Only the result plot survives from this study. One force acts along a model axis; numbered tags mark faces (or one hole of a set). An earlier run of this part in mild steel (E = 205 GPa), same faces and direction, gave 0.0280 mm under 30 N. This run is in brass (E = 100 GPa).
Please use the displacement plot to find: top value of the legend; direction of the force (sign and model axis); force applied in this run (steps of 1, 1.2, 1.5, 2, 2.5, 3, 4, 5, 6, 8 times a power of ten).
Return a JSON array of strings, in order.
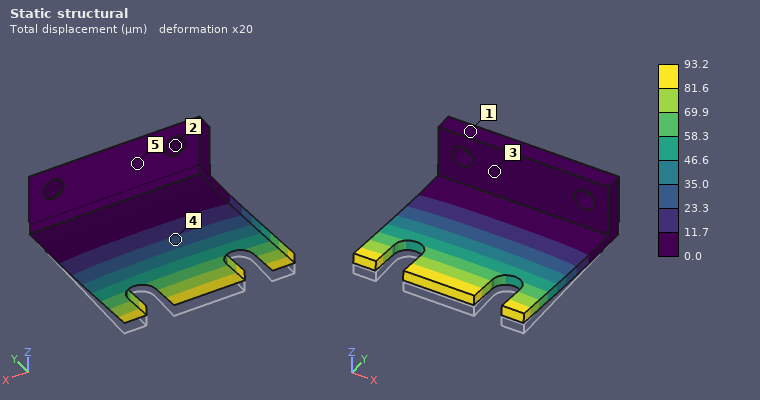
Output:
["93.2 µm", "+Z", "50 N"]
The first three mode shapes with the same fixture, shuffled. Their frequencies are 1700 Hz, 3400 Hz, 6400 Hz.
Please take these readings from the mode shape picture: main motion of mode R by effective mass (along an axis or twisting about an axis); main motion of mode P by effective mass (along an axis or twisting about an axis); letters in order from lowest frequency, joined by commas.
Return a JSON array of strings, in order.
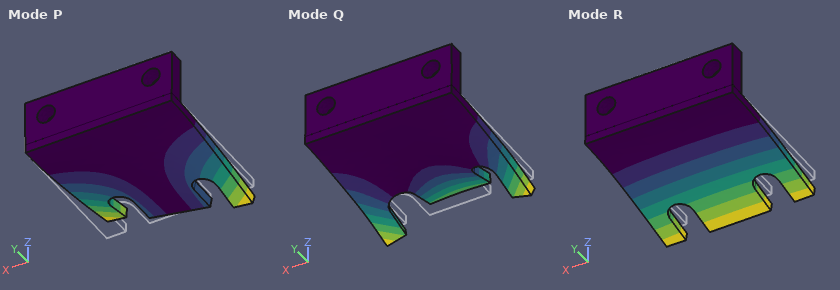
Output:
["along Z", "twisting about Y", "R, P, Q"]
